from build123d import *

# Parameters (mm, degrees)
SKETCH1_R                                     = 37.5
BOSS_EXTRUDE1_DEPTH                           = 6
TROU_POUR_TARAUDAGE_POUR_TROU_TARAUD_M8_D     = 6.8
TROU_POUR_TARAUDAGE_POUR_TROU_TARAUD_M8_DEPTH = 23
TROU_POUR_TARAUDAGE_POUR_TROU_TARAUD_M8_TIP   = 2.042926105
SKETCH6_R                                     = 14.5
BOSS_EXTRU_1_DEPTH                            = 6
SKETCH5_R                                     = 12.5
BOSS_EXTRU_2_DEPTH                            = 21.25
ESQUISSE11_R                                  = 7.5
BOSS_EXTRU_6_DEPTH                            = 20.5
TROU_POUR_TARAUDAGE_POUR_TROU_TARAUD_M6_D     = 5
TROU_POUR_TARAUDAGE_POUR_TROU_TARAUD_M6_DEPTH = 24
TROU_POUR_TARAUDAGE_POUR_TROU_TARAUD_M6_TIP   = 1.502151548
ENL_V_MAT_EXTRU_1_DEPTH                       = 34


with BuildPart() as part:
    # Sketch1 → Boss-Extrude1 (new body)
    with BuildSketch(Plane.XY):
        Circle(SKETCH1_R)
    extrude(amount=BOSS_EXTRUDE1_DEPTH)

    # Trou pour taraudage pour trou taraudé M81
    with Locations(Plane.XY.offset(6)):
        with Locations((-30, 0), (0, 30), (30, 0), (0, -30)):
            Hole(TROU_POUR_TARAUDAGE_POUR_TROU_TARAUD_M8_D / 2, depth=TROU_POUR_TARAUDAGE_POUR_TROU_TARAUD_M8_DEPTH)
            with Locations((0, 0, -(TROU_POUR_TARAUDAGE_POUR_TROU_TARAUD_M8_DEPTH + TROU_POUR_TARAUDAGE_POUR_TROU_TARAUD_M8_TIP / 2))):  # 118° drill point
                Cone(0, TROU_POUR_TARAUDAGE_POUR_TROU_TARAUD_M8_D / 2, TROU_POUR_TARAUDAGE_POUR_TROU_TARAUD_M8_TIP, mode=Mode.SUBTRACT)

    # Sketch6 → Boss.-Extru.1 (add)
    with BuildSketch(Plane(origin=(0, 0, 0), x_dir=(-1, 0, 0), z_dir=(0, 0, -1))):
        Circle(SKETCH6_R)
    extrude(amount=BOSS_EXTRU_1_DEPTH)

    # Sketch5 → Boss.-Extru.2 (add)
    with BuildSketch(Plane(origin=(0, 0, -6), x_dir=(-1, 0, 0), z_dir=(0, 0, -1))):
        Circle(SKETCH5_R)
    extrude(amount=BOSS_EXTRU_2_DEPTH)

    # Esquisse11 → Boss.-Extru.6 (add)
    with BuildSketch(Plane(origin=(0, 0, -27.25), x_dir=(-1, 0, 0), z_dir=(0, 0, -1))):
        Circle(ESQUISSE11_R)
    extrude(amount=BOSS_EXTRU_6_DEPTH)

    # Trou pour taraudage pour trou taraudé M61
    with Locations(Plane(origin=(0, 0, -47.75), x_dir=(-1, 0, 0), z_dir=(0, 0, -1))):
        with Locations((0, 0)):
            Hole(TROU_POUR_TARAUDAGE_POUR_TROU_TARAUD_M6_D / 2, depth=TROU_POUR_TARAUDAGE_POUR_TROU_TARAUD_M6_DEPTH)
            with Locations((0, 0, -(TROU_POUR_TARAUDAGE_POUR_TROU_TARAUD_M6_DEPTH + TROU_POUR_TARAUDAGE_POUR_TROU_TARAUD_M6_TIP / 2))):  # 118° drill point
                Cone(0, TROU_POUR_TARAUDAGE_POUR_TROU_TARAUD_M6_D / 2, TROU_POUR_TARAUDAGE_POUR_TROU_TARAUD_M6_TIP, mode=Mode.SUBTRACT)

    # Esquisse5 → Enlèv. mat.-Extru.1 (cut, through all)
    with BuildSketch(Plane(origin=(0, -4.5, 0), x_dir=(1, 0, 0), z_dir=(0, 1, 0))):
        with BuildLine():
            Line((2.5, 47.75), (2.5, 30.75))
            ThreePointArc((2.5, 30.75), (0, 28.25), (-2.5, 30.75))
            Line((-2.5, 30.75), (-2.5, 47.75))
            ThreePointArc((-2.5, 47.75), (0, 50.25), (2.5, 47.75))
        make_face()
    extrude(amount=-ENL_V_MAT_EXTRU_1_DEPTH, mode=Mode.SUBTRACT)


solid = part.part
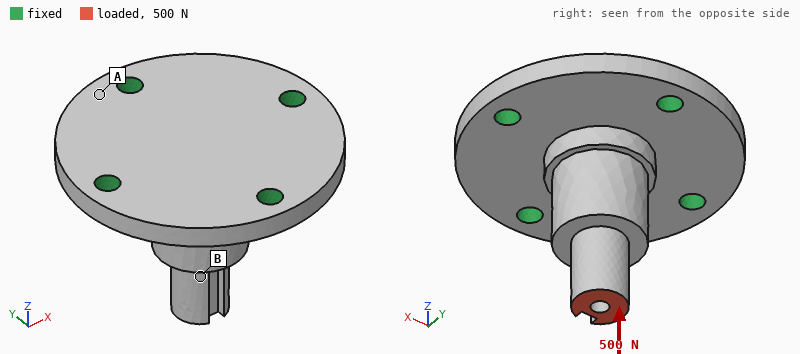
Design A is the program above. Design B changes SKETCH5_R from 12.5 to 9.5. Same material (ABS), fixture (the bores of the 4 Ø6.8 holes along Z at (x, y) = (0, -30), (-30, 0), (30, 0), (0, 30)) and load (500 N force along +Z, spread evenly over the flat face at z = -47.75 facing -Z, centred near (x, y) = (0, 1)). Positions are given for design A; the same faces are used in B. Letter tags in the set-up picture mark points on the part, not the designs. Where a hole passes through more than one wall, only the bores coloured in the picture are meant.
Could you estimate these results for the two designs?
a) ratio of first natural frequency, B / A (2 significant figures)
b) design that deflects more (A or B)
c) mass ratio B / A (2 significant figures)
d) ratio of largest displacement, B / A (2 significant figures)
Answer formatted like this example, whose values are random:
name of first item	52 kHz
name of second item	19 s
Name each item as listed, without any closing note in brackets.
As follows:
ratio of first natural frequency, B / A	0.94
design that deflects more	B
mass ratio B / A	0.90
ratio of largest displacement, B / A	1.1
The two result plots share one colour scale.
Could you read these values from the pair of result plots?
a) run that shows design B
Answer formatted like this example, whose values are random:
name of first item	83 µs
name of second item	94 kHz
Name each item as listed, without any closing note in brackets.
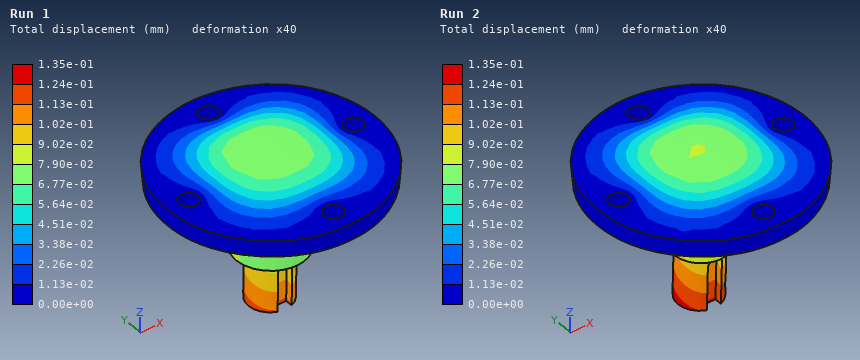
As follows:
run that shows design B	Run 2
